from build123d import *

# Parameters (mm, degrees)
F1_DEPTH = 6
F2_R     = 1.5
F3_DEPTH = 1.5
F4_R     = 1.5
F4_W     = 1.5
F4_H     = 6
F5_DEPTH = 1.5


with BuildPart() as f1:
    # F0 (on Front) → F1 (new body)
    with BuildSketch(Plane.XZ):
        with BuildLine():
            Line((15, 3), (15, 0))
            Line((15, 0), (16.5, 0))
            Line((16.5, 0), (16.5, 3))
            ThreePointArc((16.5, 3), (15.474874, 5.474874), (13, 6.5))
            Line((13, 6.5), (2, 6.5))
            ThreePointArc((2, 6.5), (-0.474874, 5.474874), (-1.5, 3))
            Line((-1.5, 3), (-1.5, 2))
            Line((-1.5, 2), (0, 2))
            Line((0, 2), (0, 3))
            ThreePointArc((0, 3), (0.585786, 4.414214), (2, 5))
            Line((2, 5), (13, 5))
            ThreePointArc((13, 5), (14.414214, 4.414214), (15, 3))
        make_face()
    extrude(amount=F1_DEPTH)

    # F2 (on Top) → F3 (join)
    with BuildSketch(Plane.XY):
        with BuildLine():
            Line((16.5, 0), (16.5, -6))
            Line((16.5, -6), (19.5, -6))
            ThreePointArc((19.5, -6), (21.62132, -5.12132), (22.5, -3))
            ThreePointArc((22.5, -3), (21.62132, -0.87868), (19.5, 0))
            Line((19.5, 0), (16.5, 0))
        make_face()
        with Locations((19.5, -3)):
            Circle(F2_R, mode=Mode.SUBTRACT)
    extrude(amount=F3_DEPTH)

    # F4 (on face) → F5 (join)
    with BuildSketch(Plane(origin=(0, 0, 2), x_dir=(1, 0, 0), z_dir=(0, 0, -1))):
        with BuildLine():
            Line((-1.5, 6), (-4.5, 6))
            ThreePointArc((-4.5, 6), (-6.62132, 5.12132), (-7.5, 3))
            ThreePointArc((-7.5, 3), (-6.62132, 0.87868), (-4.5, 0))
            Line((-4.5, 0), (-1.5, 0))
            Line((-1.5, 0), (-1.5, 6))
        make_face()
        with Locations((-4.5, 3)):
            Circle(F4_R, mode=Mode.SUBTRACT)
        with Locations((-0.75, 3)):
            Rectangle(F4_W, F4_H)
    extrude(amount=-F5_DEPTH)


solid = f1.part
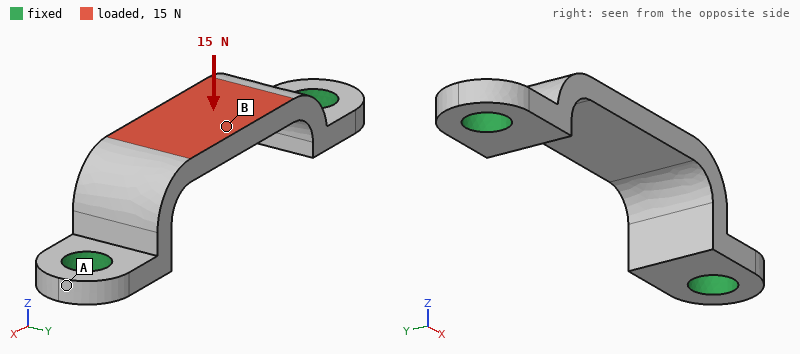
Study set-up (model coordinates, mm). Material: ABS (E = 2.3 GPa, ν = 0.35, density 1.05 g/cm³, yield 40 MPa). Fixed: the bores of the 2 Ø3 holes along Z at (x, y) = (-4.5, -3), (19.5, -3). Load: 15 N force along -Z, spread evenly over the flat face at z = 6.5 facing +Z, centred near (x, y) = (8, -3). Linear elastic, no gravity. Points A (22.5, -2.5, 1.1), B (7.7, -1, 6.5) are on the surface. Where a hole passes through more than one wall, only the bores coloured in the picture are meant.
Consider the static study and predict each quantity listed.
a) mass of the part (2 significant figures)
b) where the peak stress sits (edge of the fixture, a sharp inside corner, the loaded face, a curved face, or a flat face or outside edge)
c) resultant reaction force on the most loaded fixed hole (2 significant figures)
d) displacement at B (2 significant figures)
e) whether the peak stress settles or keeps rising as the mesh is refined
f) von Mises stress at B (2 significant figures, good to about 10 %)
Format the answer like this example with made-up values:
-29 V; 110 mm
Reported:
0.30 g; edge of the fixture; 12 N; 69 µm; keeps rising; 7.1 MPa
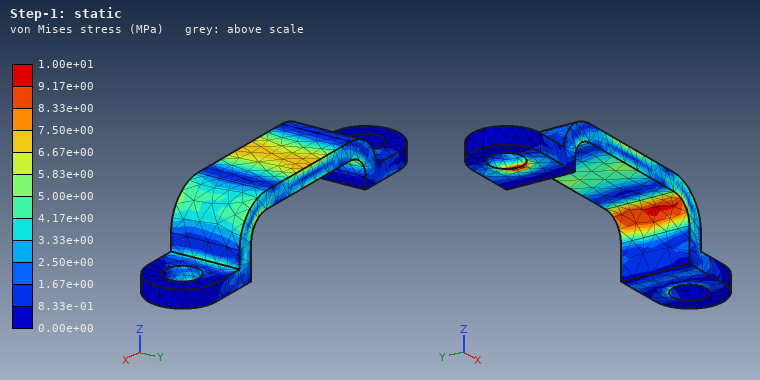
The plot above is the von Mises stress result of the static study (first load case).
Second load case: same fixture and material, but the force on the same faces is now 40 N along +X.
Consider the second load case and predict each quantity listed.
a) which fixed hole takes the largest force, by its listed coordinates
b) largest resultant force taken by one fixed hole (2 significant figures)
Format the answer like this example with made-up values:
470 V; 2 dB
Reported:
(-4.5, -3); 28 N
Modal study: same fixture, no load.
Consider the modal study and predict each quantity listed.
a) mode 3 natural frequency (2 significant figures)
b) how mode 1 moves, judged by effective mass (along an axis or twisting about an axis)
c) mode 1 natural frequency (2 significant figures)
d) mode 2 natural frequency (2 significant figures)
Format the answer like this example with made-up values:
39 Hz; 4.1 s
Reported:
9100 Hz; along Y; 6200 Hz; 7000 Hz
